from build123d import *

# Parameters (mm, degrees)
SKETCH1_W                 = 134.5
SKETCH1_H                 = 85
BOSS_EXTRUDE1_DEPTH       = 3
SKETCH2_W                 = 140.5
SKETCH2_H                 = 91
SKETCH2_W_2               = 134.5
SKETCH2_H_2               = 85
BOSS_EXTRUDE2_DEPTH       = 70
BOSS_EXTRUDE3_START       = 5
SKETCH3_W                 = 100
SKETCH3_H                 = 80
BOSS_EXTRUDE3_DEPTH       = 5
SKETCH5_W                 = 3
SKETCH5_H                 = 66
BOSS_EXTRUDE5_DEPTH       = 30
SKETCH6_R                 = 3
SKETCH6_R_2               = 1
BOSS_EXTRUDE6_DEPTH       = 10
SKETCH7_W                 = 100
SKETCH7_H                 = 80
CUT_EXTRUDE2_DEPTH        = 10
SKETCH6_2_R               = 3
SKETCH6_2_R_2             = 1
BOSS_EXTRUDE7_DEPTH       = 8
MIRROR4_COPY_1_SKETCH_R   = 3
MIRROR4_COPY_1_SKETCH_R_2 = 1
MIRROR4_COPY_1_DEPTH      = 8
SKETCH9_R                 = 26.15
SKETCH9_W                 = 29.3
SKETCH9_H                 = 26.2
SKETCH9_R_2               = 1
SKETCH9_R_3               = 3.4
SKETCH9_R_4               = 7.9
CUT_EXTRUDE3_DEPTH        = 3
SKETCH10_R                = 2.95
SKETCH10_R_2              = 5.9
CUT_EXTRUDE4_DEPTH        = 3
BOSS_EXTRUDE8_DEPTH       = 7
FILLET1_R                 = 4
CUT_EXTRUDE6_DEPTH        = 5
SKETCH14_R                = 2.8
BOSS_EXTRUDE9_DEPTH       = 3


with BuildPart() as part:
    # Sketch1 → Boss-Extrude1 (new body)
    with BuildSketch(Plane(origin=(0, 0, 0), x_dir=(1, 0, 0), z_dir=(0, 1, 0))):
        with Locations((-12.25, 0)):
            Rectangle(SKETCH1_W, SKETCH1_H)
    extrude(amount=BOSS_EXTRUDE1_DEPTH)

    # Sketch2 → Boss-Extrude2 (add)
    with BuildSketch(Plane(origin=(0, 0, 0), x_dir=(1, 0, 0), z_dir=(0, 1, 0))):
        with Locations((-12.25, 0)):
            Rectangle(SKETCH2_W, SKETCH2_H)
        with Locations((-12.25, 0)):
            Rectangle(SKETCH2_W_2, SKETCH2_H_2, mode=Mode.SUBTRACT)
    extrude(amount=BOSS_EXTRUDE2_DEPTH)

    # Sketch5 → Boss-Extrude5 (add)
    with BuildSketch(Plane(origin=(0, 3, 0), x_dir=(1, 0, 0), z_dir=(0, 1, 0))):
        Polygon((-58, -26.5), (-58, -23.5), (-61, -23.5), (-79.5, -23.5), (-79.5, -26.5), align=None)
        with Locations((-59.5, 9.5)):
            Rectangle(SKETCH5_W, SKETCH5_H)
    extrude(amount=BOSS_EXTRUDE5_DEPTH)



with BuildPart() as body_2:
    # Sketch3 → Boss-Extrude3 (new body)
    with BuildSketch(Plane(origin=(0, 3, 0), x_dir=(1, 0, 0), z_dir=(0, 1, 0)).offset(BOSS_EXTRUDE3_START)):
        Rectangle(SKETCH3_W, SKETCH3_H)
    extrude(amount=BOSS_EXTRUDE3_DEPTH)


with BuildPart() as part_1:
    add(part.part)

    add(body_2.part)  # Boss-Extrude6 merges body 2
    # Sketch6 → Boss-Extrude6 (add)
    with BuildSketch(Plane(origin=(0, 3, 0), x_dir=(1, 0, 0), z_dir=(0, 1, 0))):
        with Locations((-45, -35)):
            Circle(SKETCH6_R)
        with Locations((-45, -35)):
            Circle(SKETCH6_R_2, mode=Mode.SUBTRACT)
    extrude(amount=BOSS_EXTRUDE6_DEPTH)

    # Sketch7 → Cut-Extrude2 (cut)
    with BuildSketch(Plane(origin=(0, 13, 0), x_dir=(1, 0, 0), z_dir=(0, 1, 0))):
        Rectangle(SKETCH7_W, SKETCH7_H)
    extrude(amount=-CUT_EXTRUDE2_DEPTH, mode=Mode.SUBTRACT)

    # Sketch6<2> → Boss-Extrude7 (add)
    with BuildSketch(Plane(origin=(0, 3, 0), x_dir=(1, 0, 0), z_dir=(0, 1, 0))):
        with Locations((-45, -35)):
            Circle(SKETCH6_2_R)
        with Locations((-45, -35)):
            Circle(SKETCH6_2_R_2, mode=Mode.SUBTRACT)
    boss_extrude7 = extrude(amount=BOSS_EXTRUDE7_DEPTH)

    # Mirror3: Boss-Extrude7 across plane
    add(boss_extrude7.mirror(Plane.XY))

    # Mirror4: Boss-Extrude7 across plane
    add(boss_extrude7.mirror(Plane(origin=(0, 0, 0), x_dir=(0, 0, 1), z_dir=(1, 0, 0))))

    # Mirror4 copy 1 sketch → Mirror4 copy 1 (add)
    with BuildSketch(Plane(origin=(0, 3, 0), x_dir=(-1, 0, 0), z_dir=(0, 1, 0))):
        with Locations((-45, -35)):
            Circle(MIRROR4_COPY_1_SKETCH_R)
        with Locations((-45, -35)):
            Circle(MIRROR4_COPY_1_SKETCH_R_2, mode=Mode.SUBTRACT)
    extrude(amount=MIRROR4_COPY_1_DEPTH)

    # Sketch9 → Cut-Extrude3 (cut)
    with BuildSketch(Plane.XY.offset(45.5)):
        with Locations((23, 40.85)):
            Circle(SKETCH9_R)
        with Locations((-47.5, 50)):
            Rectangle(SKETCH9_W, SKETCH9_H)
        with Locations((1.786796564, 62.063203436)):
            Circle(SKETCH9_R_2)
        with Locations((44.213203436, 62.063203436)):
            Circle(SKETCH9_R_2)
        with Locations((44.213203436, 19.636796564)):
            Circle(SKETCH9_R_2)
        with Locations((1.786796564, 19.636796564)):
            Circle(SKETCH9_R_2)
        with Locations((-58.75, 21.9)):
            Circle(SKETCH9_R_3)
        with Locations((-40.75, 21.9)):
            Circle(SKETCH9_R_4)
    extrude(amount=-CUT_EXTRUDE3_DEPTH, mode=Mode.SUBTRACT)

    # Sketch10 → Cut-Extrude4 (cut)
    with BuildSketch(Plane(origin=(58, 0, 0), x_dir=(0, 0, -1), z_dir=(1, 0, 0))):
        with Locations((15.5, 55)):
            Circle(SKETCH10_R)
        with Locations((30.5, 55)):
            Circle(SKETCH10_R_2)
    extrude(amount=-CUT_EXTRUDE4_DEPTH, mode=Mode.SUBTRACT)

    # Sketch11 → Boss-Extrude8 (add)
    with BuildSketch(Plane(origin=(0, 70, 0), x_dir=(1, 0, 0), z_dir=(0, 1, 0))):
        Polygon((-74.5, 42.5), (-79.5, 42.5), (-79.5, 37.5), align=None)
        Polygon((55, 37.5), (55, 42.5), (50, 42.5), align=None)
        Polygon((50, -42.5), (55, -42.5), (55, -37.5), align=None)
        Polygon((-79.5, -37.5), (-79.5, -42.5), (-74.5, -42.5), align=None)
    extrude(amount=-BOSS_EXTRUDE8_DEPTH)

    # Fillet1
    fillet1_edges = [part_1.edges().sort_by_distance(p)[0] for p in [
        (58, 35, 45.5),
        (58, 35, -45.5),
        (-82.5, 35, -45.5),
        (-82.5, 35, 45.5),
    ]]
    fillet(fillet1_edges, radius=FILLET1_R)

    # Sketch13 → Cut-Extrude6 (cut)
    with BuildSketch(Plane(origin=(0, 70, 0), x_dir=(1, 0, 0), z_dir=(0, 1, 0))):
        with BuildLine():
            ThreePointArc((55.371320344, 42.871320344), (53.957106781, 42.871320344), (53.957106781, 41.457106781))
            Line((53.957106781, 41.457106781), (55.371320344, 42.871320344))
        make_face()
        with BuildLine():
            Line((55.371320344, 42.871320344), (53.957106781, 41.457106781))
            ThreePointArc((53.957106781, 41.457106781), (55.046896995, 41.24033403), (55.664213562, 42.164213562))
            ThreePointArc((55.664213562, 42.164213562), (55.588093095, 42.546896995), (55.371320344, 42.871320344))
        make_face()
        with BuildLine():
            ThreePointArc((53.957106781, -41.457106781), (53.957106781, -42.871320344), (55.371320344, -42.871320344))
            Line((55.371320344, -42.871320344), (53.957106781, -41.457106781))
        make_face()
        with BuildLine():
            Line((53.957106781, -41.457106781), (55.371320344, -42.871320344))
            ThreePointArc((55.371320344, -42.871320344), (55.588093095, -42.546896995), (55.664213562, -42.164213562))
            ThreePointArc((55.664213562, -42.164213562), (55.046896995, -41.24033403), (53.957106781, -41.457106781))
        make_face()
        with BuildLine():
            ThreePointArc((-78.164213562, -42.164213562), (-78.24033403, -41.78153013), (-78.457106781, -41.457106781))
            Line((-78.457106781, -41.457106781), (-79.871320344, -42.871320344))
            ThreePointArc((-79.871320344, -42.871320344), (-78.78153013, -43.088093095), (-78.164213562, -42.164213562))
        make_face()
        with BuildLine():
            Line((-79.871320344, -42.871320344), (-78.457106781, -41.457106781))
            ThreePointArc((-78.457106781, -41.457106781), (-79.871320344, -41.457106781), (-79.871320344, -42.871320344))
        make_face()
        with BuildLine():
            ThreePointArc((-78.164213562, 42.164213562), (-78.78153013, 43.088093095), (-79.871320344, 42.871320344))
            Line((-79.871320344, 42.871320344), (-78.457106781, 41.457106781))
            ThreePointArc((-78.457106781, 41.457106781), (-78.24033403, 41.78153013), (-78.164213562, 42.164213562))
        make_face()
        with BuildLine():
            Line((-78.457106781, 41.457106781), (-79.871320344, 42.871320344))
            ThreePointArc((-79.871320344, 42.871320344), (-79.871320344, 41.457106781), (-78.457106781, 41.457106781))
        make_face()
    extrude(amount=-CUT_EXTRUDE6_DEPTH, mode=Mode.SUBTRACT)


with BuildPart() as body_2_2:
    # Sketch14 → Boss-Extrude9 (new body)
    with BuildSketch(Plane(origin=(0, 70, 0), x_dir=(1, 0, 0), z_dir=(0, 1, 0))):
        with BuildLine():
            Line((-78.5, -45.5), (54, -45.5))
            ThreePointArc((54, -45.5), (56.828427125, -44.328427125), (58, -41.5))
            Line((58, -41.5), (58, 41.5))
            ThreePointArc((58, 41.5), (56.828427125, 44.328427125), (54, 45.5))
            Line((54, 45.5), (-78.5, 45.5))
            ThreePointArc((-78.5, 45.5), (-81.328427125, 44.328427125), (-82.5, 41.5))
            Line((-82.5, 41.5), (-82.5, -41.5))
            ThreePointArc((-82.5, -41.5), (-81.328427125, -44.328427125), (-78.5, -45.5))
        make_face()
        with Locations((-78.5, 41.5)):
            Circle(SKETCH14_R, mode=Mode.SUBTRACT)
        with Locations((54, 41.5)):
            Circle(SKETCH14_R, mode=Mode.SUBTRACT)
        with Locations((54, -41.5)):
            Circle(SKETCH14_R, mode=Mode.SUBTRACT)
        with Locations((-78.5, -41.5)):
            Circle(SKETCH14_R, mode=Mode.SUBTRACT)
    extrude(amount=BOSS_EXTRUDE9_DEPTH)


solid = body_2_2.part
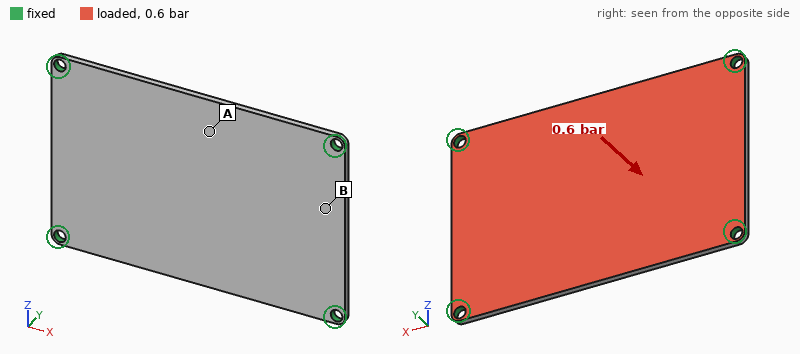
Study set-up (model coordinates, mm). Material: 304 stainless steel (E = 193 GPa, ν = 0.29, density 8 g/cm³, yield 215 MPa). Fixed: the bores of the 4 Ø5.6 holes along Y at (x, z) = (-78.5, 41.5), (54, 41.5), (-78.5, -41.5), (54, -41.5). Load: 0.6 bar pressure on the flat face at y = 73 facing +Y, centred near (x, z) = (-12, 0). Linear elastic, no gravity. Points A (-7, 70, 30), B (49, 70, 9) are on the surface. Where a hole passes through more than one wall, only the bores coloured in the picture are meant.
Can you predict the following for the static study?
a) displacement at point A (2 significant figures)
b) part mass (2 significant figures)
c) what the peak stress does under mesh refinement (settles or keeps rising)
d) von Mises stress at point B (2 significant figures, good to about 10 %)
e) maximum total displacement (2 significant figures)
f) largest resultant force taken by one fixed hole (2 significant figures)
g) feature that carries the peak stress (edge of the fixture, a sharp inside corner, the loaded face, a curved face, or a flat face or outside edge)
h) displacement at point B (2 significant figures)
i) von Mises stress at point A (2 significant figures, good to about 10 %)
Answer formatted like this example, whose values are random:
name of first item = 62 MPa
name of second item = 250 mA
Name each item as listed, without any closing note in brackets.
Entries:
displacement at point A = 0.17 mm
part mass = 300 g
what the peak stress does under mesh refinement = keeps rising
von Mises stress at point B = 18 MPa
maximum total displacement = 0.18 mm
largest resultant force taken by one fixed hole = 190 N
feature that carries the peak stress = edge of the fixture
displacement at point B = 0.037 mm
von Mises stress at point A = 35 MPa
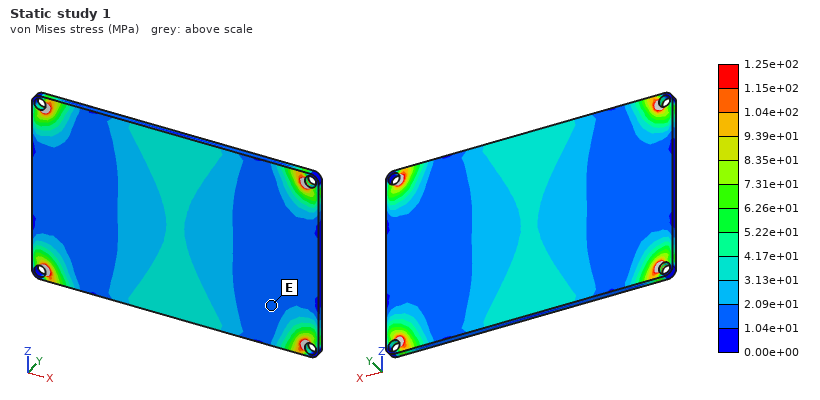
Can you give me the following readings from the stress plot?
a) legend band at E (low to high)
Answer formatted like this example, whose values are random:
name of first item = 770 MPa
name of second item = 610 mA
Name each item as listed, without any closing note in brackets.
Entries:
legend band at E = 1.04e+01 to 2.09e+01 MPa
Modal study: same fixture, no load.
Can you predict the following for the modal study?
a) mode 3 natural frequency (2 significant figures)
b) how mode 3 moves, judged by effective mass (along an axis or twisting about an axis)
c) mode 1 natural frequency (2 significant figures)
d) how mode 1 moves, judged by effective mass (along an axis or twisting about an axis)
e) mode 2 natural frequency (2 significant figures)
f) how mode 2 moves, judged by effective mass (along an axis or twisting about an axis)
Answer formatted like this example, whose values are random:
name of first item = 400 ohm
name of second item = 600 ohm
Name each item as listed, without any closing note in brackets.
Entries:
mode 3 natural frequency = 1800 Hz
how mode 3 moves, judged by effective mass = twisting about Z
mode 1 natural frequency = 690 Hz
how mode 1 moves, judged by effective mass = along Y
mode 2 natural frequency = 1200 Hz
how mode 2 moves, judged by effective mass = twisting about X
